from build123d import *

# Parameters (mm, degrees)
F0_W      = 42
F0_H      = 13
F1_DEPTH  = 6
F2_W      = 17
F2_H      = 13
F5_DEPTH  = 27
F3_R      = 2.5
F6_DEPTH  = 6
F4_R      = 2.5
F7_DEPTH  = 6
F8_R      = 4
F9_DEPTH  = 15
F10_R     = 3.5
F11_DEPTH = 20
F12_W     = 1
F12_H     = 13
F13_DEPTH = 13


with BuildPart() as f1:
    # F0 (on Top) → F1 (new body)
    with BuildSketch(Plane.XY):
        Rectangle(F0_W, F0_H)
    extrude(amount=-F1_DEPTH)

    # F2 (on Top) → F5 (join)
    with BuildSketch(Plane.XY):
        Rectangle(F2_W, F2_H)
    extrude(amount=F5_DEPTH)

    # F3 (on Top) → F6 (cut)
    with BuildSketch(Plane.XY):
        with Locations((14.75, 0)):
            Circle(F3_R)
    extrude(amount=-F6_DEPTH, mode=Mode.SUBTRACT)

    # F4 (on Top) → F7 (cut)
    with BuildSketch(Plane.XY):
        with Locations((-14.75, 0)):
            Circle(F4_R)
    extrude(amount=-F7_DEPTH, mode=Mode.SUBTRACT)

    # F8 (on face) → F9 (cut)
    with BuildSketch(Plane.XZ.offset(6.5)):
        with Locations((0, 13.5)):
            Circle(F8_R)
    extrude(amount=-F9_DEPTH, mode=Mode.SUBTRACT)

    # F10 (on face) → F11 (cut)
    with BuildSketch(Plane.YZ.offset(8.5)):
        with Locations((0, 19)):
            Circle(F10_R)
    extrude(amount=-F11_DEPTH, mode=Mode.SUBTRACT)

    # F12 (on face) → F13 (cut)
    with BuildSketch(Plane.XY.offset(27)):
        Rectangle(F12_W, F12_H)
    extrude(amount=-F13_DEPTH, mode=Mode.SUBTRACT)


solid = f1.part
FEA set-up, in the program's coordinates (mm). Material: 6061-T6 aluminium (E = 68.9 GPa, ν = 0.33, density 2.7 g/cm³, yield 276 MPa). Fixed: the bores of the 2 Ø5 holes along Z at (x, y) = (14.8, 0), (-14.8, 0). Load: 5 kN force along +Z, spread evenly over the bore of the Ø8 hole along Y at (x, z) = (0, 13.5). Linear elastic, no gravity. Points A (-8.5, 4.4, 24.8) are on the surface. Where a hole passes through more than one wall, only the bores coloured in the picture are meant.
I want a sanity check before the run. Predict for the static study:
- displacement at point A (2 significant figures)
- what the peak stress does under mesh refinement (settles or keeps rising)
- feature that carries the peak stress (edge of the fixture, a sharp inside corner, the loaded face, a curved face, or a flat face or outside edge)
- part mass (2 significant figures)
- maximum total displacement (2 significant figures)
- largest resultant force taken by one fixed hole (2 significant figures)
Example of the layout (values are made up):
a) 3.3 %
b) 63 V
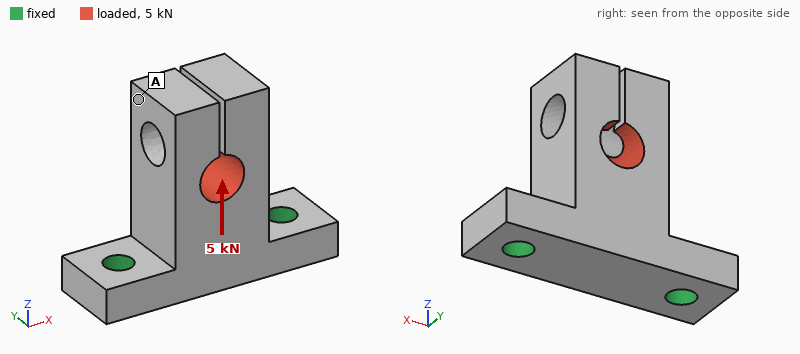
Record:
a) 53 µm
b) keeps rising
c) edge of the fixture
d) 21 g
e) 77 µm
f) 2.7 kN
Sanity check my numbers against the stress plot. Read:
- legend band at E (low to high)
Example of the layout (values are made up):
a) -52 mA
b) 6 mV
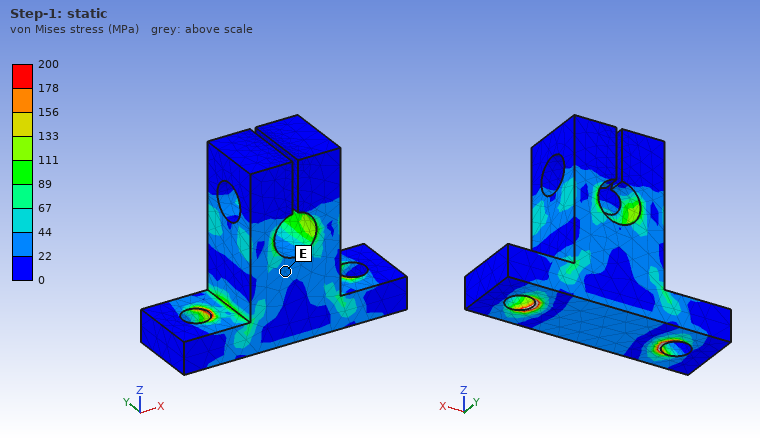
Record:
a) 22 to 44 MPa
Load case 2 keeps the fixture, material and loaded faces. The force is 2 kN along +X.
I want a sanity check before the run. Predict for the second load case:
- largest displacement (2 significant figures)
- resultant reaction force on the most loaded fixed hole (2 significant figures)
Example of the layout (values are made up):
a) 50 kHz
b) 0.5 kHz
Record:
a) 66 µm
b) 1.7 kN
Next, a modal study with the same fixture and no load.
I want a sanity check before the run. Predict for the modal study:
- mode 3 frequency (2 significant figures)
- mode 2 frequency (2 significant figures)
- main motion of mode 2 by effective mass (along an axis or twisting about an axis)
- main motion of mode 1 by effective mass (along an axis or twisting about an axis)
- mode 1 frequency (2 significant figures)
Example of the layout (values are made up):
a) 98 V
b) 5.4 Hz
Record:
a) 8200 Hz
b) 7300 Hz
c) along X
d) along Y
e) 5300 Hz
